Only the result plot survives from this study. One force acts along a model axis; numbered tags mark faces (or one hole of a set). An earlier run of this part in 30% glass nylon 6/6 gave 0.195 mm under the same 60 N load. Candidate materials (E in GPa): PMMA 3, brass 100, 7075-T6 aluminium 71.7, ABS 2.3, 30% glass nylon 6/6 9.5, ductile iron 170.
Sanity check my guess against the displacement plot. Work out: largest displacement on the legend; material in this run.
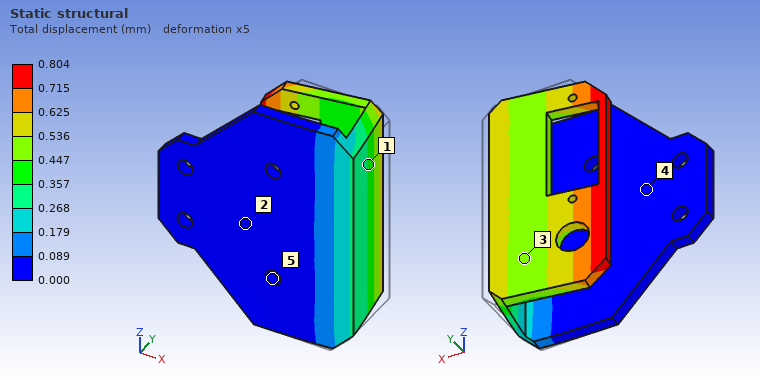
0.804 mm
ABS
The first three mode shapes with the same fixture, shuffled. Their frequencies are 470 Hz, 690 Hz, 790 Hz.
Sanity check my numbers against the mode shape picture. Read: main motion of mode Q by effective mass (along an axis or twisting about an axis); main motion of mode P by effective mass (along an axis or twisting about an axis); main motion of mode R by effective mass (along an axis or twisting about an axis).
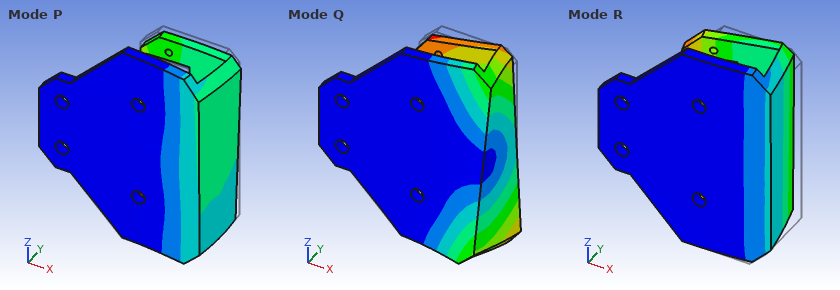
along Z
along Y
along X
